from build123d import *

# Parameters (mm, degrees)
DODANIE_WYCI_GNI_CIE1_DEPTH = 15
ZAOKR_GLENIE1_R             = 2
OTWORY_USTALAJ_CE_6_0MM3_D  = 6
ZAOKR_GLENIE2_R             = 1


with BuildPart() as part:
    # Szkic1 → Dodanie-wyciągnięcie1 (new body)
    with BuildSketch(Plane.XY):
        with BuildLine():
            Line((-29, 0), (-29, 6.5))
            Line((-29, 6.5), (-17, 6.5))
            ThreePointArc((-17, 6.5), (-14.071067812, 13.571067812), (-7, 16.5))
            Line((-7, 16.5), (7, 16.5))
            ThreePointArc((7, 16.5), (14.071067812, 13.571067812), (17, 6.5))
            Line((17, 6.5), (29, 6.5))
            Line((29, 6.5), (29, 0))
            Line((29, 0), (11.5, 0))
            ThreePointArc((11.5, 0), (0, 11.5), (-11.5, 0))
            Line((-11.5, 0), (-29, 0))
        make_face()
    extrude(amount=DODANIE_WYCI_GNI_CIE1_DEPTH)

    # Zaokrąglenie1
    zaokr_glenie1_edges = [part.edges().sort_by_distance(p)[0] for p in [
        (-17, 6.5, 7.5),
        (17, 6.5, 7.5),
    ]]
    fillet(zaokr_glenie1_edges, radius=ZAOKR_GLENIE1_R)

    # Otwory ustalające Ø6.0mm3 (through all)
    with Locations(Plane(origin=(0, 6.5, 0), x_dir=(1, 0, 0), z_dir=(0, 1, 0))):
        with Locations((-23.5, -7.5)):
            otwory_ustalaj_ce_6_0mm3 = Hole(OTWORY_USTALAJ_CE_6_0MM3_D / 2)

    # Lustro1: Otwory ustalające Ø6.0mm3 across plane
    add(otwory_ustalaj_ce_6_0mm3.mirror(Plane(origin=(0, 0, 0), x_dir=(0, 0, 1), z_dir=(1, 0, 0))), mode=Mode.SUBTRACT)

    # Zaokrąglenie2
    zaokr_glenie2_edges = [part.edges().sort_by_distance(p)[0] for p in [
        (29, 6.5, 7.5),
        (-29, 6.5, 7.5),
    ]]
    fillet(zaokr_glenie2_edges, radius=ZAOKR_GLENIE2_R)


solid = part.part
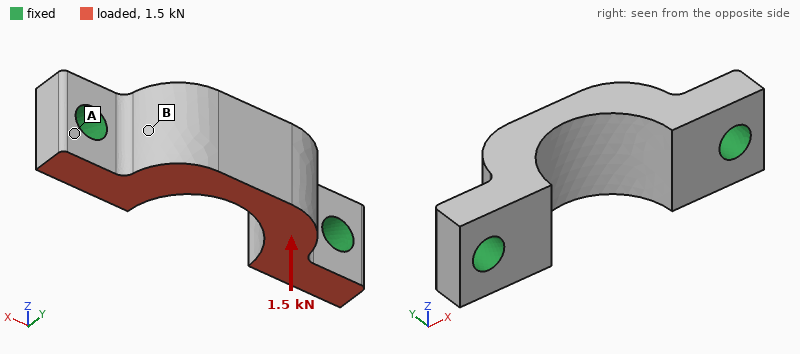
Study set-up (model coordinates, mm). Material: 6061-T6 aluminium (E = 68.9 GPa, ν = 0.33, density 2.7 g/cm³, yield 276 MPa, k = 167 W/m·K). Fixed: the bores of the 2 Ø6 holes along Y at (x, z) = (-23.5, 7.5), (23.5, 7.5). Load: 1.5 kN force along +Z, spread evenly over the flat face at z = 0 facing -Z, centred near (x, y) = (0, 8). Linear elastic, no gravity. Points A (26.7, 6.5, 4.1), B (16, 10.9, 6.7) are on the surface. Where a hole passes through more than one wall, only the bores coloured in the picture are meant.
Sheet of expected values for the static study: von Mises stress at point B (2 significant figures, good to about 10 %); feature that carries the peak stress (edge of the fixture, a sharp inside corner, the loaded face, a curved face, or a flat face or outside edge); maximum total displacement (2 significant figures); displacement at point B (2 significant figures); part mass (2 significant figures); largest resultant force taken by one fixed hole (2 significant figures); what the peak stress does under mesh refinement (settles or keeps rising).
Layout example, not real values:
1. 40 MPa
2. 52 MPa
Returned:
1. 13 MPa
2. edge of the fixture
3. 18 µm
4. 8.7 µm
5. 18 g
6. 750 N
7. keeps rising
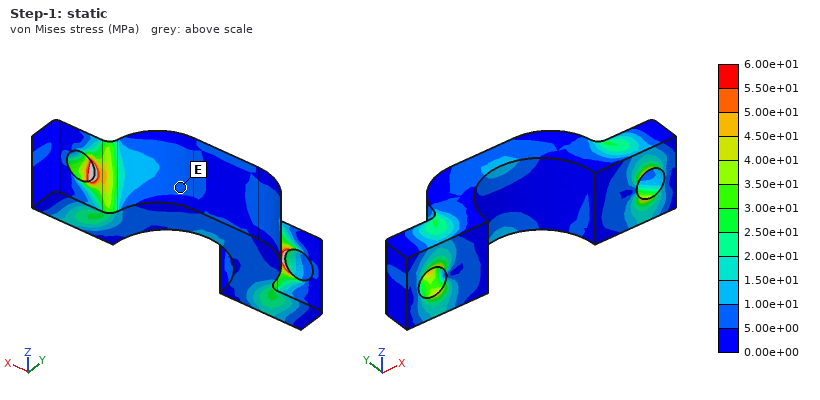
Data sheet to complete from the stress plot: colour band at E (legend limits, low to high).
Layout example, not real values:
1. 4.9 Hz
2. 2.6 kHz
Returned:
1. 5.00e+00 to 1.00e+01 MPa
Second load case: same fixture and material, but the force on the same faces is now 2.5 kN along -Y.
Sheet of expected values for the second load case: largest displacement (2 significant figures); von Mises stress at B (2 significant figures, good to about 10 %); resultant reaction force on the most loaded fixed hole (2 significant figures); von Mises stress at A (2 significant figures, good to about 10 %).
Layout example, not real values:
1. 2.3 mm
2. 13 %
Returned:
1. 33 µm
2. 18 MPa
3. 1.4 kN
4. 20 MPa
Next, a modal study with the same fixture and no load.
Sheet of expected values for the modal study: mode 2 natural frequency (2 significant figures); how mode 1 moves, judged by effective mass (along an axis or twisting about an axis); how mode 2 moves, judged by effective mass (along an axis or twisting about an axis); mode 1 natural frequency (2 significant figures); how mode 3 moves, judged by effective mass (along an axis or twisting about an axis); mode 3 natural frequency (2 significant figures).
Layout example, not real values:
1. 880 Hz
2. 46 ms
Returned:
1. 24 kHz
2. along Z
3. along Y
4. 13 kHz
5. along X
6. 26 kHz
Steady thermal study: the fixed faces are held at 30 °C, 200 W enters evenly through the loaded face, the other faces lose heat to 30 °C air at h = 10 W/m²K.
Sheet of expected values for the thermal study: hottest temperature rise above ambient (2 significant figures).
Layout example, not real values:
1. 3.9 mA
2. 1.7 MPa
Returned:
1. 70 K
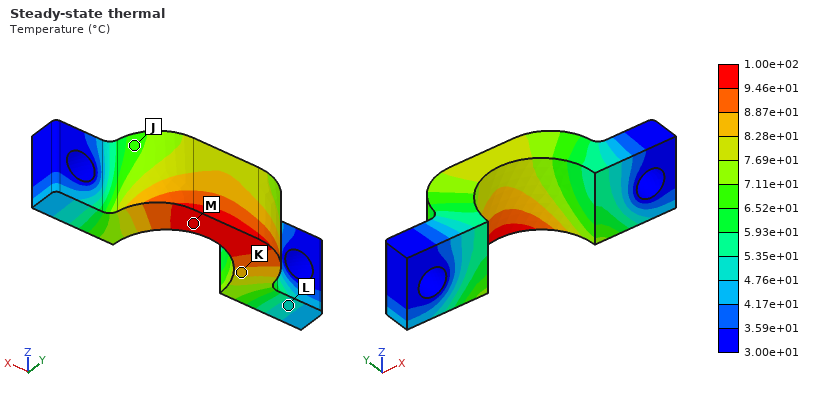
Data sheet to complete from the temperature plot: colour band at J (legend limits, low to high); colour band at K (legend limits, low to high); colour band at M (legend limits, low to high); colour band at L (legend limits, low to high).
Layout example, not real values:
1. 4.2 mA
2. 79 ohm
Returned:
1. 6.52e+01 to 7.11e+01 °C
2. 8.28e+01 to 8.87e+01 °C
3. 9.46e+01 to 1.00e+02 °C
4. 4.76e+01 to 5.35e+01 °C
